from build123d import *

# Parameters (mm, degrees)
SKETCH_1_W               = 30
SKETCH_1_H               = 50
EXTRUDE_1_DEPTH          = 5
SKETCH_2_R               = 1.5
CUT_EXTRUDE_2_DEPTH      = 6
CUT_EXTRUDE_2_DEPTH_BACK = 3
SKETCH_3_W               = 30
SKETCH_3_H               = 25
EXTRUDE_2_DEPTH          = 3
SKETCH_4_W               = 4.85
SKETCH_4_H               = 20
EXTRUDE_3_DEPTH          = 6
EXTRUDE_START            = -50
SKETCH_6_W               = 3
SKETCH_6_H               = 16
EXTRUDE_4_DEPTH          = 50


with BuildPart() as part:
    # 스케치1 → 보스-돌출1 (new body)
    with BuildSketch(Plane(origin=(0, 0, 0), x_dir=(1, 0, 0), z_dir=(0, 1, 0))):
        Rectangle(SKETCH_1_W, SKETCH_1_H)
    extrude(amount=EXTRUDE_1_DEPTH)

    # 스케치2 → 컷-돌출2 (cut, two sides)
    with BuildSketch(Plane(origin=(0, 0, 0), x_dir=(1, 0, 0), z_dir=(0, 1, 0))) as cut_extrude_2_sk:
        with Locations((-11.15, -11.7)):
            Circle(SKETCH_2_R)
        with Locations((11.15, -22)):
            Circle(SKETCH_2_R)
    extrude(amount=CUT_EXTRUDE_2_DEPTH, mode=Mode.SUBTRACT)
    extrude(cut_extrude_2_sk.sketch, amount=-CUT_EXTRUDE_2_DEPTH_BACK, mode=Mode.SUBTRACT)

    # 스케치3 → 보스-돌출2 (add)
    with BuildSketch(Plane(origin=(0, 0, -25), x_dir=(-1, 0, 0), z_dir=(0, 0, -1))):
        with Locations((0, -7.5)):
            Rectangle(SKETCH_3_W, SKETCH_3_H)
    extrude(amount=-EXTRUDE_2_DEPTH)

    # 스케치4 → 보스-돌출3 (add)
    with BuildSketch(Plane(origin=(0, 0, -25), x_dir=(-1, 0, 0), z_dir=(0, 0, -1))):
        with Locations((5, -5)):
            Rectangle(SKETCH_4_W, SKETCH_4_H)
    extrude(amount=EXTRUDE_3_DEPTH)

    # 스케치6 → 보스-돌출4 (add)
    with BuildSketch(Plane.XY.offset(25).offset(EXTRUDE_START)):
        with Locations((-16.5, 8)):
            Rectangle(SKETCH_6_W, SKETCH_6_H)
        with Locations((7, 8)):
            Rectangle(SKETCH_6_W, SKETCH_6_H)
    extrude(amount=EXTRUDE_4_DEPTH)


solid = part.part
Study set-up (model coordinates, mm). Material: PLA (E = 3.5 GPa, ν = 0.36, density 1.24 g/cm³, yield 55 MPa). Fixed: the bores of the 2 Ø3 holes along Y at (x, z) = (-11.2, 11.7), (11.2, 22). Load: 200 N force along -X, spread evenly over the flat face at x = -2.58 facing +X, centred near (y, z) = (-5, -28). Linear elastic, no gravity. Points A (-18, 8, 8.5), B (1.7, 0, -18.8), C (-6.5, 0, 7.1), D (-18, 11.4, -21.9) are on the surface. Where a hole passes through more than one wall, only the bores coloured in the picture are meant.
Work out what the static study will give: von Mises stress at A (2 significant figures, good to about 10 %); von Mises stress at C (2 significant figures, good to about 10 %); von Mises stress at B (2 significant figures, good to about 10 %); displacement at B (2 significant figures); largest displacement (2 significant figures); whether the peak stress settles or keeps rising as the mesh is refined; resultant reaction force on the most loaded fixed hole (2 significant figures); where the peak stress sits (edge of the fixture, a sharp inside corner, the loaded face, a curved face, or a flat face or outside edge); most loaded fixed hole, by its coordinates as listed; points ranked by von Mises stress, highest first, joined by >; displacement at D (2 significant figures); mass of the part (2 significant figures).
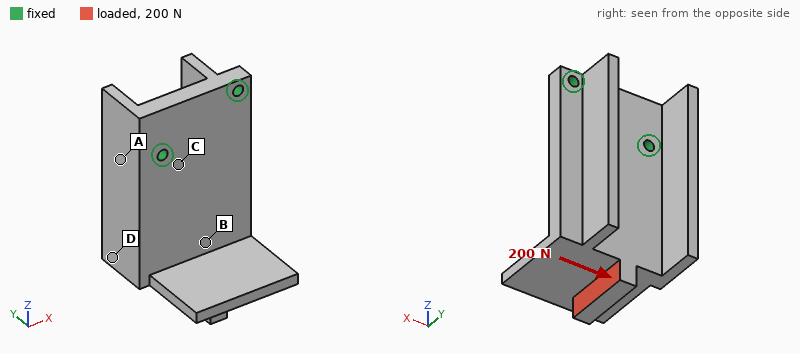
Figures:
4.4 MPa
11 MPa
8.6 MPa
0.23 mm
0.76 mm
keeps rising
400 N
edge of the fixture
(-11.2, 11.7)
C > B > A > D
0.21 mm
17 g
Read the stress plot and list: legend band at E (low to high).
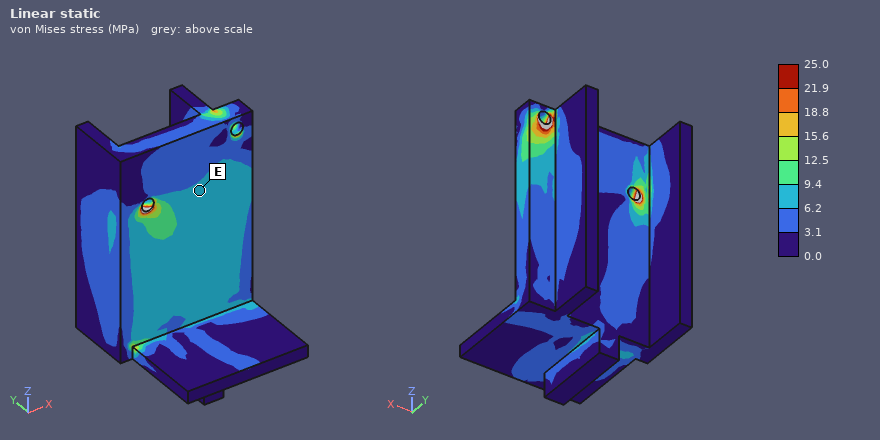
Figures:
6.2 to 9.4 MPa
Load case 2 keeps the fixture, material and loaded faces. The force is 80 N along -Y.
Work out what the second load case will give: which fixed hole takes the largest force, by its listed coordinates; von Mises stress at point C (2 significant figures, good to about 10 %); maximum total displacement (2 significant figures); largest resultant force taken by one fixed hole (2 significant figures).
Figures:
(-11.2, 11.7)
9.5 MPa
0.84 mm
96 N
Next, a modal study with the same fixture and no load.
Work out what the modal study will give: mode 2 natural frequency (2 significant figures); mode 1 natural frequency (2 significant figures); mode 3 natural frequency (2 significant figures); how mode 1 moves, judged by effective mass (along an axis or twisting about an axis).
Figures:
1200 Hz
710 Hz
2000 Hz
along Y
